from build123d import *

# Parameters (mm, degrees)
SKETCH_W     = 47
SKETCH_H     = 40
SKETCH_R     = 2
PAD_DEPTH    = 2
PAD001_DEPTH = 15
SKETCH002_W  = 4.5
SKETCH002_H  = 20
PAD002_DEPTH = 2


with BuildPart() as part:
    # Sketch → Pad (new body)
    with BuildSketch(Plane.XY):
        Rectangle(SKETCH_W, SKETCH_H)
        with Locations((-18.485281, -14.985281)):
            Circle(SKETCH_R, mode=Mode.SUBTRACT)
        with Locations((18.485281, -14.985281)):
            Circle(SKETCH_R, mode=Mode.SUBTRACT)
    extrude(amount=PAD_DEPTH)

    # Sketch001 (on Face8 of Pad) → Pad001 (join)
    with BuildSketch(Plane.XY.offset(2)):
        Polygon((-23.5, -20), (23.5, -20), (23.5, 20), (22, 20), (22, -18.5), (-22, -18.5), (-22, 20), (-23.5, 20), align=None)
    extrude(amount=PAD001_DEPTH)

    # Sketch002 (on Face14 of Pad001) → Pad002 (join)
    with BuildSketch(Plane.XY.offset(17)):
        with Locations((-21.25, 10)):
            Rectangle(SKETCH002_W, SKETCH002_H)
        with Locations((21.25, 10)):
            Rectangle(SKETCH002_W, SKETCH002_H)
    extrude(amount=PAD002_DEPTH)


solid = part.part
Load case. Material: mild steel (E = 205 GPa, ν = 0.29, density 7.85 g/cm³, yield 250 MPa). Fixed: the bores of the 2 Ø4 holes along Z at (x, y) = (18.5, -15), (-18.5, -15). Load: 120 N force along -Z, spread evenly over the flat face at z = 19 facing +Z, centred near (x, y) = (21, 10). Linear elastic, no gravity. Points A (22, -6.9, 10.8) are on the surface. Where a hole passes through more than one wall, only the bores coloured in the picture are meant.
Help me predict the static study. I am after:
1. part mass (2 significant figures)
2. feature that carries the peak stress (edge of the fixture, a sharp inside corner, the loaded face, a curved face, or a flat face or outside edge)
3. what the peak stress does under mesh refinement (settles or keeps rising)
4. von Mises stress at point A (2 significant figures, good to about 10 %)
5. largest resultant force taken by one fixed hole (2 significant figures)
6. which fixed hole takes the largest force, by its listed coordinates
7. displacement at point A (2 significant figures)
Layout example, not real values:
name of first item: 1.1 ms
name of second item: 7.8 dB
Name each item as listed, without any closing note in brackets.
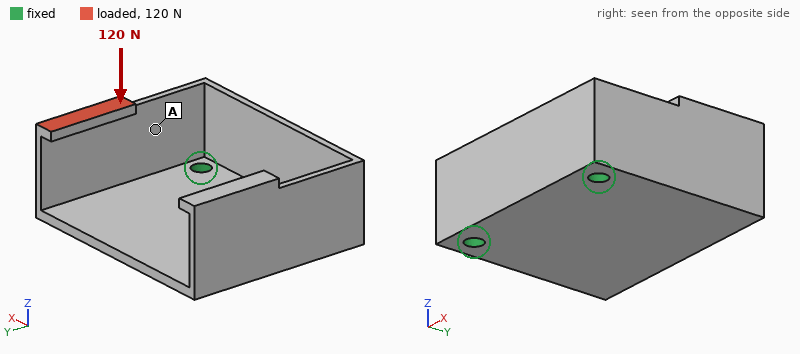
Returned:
part mass: 54 g
feature that carries the peak stress: edge of the fixture
what the peak stress does under mesh refinement: keeps rising
von Mises stress at point A: 12 MPa
largest resultant force taken by one fixed hole: 110 N
which fixed hole takes the largest force, by its listed coordinates: (18.5, -15)
displacement at point A: 20 µm
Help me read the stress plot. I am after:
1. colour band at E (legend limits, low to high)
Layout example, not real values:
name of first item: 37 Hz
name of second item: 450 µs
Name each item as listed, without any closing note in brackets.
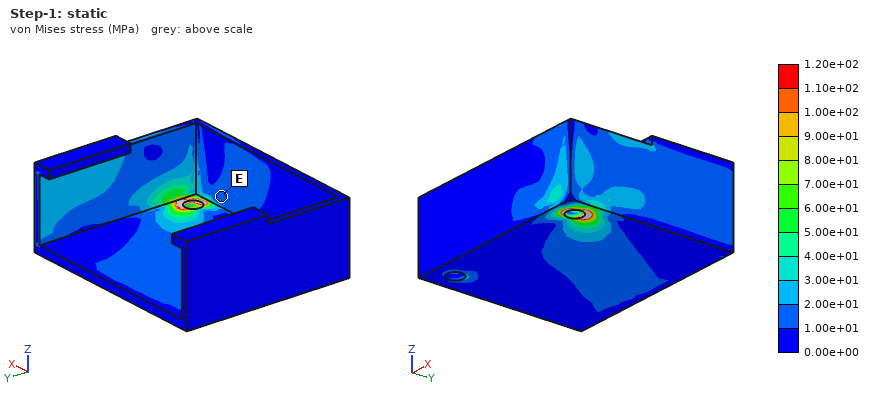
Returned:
colour band at E: 1.00e+01 to 2.00e+01 MPa
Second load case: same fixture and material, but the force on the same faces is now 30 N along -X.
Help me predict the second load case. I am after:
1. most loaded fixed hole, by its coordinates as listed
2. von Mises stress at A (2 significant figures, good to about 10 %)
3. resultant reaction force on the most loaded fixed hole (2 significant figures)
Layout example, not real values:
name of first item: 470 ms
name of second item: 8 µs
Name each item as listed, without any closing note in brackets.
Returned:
most loaded fixed hole, by its coordinates as listed: (-18.5, -15)
von Mises stress at A: 25 MPa
resultant reaction force on the most loaded fixed hole: 31 N
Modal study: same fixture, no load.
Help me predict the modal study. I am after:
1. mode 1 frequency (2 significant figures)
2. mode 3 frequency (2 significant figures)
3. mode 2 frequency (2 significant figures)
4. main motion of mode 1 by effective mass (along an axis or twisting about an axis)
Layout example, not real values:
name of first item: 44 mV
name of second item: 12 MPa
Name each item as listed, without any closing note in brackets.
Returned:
mode 1 frequency: 2000 Hz
mode 3 frequency: 2600 Hz
mode 2 frequency: 2500 Hz
main motion of mode 1 by effective mass: along Z
